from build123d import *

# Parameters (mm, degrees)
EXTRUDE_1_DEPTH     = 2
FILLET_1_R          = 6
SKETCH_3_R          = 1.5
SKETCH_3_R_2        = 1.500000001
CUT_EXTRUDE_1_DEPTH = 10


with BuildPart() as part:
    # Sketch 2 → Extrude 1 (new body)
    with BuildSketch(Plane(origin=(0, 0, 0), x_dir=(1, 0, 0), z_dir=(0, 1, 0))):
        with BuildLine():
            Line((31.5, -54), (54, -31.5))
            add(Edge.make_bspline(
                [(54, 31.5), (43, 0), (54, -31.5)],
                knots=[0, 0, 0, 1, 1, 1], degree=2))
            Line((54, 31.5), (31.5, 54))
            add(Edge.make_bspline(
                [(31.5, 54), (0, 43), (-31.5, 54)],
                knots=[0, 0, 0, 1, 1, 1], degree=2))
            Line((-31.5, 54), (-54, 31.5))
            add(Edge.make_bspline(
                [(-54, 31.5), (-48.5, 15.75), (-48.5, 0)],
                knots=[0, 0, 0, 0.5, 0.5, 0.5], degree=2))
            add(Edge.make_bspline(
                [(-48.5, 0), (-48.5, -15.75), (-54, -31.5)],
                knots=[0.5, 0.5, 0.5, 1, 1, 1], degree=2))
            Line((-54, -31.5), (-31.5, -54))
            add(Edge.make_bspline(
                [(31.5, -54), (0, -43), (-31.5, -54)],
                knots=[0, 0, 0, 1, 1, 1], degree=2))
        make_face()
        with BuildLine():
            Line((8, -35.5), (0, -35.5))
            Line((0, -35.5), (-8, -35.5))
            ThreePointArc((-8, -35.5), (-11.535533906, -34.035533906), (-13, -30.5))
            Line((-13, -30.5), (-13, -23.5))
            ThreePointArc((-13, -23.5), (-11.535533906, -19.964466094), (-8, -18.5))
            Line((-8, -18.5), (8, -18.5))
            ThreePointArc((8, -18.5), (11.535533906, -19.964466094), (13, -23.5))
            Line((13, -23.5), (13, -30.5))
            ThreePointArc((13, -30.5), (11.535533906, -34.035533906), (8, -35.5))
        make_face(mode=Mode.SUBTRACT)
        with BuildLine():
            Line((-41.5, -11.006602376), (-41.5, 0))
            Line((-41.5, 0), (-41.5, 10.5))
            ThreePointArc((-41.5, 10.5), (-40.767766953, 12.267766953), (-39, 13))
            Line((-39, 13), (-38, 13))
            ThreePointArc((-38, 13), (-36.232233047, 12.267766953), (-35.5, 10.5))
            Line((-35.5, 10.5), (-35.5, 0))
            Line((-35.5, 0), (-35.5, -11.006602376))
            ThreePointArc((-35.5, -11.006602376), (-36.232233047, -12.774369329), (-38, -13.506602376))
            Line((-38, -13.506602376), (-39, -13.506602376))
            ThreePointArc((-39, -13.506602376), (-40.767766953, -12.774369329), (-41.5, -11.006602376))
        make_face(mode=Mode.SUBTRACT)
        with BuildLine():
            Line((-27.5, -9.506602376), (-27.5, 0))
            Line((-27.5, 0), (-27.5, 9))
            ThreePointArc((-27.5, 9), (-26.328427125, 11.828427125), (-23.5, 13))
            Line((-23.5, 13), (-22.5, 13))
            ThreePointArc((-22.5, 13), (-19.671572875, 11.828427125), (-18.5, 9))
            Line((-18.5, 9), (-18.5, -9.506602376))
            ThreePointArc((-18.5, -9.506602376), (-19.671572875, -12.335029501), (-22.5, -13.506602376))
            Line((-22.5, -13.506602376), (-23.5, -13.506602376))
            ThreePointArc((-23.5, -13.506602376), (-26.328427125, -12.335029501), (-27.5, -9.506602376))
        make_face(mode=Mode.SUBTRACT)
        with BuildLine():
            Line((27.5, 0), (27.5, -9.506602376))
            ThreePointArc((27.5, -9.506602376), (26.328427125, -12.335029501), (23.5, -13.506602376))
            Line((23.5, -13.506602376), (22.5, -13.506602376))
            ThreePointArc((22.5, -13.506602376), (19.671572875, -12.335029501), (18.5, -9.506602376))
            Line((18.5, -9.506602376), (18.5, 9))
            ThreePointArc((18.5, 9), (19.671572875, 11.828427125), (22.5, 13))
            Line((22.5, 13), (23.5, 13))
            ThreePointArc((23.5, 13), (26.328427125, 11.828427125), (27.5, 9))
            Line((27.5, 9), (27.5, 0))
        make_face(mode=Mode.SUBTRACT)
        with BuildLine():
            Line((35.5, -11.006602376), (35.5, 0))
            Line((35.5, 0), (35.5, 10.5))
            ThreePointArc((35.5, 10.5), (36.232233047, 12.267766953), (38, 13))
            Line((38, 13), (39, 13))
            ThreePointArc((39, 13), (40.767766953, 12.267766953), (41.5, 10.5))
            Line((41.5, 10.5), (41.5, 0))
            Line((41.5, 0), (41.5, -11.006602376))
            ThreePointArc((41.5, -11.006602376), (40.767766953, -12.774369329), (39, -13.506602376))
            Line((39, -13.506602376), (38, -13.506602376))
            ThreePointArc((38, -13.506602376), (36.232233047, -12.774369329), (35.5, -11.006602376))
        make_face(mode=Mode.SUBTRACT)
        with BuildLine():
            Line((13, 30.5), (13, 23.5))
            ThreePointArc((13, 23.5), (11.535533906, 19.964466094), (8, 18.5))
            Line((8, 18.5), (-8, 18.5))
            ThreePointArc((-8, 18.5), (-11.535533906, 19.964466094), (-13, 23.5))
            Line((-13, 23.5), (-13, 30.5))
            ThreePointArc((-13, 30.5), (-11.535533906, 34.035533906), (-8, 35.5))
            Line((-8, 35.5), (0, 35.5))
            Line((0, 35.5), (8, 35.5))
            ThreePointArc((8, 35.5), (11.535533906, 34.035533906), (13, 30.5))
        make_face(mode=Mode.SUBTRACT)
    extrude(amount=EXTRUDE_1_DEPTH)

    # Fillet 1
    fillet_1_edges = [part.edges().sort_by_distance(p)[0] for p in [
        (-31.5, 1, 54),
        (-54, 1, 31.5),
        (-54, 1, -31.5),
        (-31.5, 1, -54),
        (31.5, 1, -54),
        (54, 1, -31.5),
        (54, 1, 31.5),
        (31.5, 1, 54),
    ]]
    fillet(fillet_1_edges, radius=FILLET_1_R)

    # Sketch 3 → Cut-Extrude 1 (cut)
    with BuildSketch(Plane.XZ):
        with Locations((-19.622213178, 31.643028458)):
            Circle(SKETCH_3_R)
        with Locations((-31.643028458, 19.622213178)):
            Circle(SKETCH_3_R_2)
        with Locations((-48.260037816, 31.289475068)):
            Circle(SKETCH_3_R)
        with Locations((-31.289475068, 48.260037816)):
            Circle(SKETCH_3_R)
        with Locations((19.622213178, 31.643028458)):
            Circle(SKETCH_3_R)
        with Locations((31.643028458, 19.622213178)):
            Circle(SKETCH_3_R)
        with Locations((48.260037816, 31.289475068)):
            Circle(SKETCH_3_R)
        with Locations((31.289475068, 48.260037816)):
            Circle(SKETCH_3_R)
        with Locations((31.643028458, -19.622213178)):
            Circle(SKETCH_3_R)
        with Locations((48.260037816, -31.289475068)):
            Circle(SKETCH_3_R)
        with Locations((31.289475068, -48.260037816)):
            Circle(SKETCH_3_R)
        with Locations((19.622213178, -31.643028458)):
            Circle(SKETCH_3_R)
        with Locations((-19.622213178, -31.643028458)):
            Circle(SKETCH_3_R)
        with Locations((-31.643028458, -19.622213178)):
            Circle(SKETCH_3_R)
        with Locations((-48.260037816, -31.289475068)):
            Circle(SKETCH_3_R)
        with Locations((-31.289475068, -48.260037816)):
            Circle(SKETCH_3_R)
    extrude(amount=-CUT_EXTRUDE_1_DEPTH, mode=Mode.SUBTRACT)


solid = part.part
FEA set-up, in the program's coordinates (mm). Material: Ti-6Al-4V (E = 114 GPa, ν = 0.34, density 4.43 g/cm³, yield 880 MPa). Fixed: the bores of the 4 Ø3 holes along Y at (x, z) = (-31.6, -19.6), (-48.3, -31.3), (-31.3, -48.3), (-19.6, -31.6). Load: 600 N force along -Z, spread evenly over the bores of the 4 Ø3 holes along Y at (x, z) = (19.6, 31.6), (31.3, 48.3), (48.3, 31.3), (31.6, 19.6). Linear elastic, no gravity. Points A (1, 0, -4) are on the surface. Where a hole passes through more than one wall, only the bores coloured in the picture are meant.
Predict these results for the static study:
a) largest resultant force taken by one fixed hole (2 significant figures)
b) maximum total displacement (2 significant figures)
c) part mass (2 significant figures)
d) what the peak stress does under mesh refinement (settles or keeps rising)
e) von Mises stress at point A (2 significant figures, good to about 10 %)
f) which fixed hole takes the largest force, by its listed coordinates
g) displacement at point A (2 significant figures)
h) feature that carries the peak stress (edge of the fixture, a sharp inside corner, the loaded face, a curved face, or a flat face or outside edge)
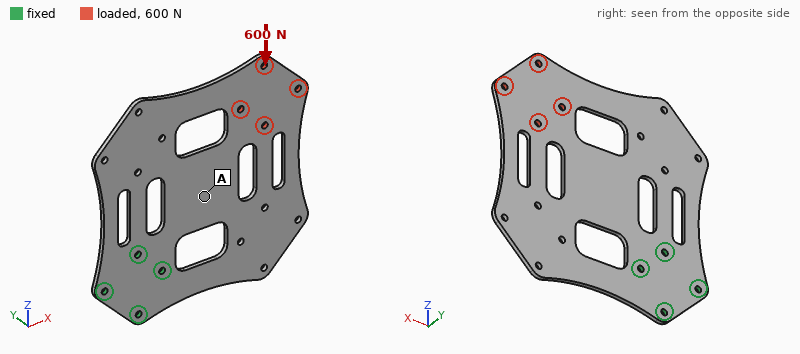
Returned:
1.0 kN
0.10 mm
71 g
keeps rising
7.6 MPa
(-19.6, -31.6)
0.038 mm
edge of the fixture
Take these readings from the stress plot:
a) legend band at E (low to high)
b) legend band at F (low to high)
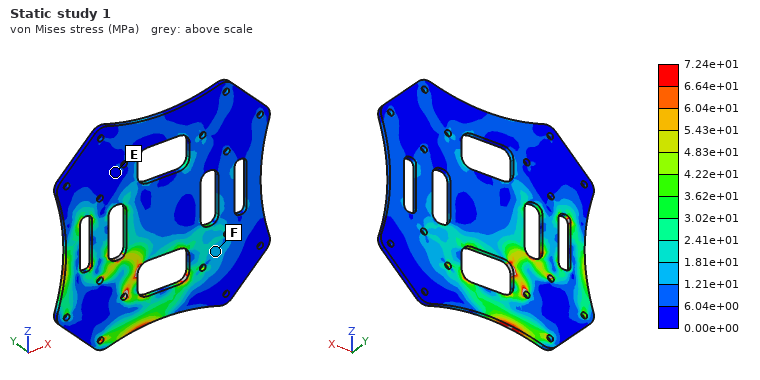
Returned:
0.00e+00 to 6.04e+00 MPa
1.21e+01 to 1.81e+01 MPa
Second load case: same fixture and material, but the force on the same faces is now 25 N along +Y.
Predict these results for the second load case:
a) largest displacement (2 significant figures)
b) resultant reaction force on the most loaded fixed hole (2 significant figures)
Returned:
1.6 mm
37 N
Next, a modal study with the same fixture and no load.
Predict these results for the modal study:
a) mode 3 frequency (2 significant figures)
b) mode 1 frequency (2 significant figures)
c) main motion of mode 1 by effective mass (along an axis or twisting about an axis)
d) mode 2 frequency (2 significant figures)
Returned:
590 Hz
160 Hz
along Y
310 Hz
